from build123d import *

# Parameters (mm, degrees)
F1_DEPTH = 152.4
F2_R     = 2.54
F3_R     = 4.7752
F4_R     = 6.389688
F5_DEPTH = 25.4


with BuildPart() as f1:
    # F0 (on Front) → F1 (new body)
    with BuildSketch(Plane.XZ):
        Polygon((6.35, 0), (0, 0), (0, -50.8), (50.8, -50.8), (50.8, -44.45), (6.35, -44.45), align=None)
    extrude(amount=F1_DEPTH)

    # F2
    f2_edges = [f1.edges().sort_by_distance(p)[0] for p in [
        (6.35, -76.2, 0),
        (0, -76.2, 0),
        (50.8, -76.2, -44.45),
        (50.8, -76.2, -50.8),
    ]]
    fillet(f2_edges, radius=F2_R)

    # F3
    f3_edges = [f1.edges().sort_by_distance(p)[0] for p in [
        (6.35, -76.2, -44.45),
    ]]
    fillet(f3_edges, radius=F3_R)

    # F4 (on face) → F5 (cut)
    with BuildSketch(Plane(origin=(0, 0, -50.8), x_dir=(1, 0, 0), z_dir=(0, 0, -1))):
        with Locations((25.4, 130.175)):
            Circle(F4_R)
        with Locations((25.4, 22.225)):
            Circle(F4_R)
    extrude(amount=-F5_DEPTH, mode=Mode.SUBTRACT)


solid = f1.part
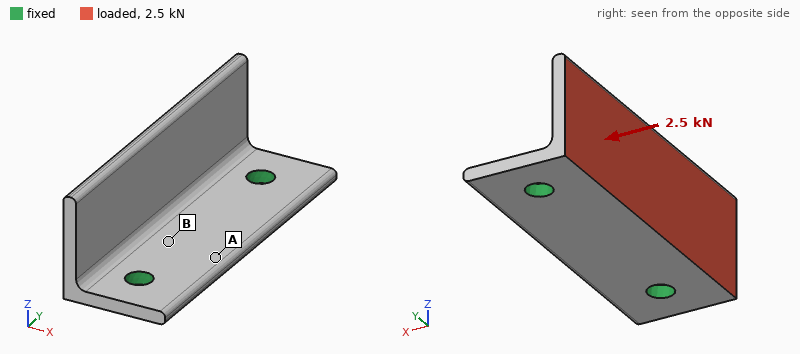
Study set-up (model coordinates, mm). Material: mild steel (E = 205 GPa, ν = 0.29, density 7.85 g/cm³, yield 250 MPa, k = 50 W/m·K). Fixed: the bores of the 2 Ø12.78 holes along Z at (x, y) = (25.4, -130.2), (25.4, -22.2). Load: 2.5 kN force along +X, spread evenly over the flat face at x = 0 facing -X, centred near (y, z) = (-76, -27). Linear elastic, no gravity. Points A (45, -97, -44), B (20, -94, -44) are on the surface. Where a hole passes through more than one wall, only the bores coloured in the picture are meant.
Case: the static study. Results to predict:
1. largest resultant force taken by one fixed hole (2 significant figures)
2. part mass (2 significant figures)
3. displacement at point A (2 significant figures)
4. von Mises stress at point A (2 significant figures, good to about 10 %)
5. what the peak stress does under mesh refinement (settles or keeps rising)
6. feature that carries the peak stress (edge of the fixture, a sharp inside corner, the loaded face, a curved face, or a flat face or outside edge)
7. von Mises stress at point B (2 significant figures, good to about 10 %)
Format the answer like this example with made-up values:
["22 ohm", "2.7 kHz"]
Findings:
["1.3 kN", "710 g", "0.017 mm", "12 MPa", "keeps rising", "edge of the fixture", "28 MPa"]
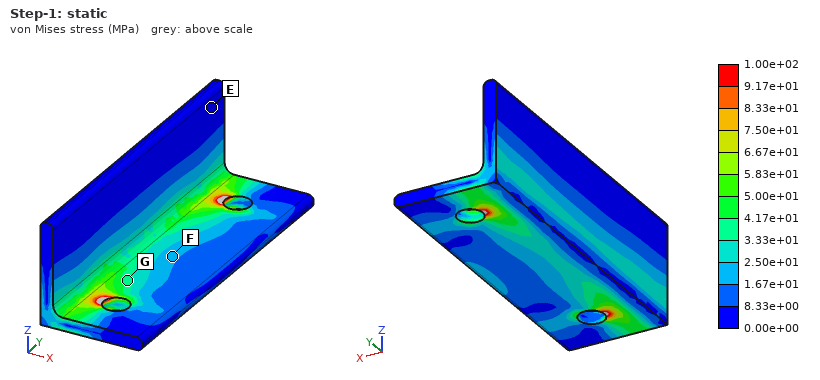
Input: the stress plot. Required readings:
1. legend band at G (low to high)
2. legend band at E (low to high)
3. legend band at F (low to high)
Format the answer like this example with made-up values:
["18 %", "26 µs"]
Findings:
["3.33e+01 to 4.17e+01 MPa", "0.00e+00 to 8.33e+00 MPa", "1.67e+01 to 2.50e+01 MPa"]
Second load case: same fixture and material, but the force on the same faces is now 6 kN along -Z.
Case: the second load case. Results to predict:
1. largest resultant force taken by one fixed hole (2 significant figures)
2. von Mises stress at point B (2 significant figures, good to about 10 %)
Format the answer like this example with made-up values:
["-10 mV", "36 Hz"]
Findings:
["3.1 kN", "34 MPa"]
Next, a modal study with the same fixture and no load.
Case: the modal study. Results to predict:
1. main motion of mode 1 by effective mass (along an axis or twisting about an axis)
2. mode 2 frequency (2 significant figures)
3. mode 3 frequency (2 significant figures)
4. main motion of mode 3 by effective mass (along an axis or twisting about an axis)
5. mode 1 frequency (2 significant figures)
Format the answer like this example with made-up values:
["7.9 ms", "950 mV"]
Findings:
["along X", "2100 Hz", "3500 Hz", "along Z", "1400 Hz"]
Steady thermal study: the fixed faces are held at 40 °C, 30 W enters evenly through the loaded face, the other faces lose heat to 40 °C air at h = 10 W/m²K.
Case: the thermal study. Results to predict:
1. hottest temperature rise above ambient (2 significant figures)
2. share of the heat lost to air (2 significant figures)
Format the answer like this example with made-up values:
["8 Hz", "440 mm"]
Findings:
["29 K", "11 %"]
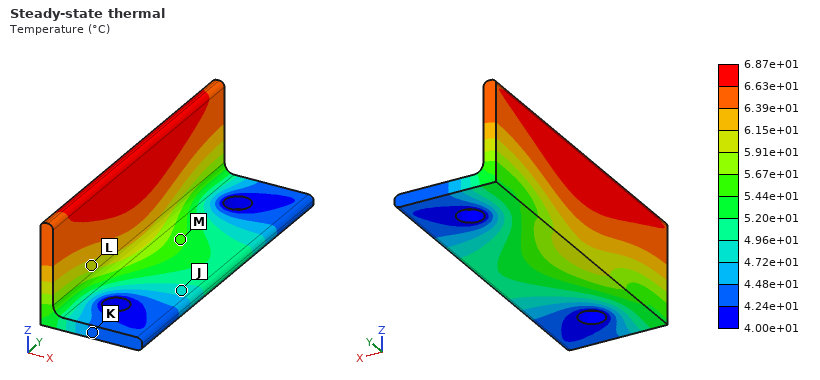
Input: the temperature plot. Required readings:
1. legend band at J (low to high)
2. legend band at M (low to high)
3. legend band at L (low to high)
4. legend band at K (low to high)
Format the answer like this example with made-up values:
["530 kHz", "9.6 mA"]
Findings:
["4.72e+01 to 4.96e+01 °C", "5.44e+01 to 5.67e+01 °C", "5.91e+01 to 6.15e+01 °C", "4.24e+01 to 4.48e+01 °C"]
